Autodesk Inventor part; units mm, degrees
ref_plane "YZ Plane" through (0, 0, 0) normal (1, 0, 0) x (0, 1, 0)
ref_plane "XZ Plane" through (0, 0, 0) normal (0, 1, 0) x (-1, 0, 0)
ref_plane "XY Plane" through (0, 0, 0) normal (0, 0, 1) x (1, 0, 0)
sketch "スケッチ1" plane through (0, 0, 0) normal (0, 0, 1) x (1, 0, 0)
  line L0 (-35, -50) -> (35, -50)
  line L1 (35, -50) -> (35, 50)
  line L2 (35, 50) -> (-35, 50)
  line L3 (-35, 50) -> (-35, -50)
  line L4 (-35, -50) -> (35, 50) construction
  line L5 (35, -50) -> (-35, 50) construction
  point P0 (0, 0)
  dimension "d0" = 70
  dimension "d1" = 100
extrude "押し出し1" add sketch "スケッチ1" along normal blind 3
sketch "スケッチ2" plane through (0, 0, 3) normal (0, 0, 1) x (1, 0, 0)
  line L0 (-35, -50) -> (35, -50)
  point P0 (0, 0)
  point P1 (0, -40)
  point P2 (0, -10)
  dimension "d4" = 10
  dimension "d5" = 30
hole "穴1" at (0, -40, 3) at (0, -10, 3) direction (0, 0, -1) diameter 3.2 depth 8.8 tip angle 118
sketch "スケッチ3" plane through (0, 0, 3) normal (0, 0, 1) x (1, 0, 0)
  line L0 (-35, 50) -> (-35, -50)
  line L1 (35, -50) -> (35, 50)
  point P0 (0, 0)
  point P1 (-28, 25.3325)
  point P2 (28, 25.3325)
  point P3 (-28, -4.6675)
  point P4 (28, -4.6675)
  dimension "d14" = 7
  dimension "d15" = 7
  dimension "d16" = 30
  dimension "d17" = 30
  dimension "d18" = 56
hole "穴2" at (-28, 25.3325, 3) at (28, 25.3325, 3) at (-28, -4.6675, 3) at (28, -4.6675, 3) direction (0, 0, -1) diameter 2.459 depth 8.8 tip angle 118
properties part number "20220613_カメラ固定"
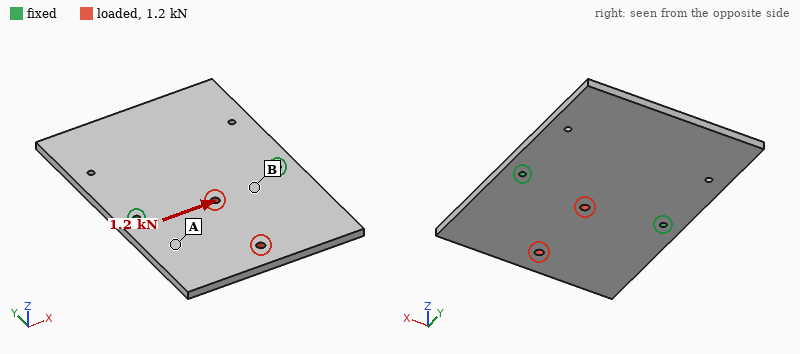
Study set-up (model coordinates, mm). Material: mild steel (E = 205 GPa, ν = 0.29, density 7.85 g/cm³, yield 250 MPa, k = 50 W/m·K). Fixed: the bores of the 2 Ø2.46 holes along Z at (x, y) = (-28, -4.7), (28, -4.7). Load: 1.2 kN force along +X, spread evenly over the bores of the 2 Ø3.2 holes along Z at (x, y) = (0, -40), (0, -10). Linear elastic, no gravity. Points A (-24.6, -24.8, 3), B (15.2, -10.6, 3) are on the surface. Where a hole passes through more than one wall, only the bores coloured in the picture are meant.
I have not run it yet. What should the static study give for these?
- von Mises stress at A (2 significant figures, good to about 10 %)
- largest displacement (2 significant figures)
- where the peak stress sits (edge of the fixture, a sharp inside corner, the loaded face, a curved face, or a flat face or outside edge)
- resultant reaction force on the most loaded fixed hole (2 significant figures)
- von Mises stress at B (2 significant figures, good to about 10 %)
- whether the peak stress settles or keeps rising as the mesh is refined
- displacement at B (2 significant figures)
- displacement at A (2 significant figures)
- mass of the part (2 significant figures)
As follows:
4.9 MPa
3.7 µm
edge of the fixture
740 N
10 MPa
keeps rising
1.1 µm
2.1 µm
160 g
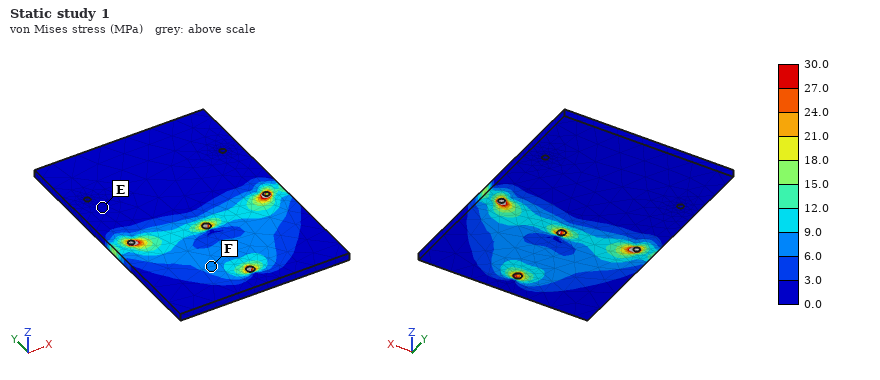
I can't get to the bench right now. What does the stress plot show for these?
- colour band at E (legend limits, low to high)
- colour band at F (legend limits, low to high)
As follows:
0.0 to 3.0 MPa
6.0 to 9.0 MPa
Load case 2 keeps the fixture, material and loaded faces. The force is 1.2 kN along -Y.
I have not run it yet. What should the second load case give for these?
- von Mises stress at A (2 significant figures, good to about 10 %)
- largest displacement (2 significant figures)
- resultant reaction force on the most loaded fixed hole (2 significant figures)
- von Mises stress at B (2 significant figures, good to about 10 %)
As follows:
5.0 MPa
2.5 µm
600 N
5.8 MPa
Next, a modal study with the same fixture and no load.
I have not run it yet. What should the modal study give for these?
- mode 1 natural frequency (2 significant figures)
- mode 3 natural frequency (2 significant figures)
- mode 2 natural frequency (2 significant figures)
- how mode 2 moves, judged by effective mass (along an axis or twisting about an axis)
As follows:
650 Hz
1700 Hz
1100 Hz
along Z
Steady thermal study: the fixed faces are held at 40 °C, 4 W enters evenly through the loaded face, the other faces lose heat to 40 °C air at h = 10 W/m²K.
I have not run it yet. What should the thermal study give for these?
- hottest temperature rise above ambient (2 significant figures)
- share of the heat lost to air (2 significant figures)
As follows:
16 K
22 %
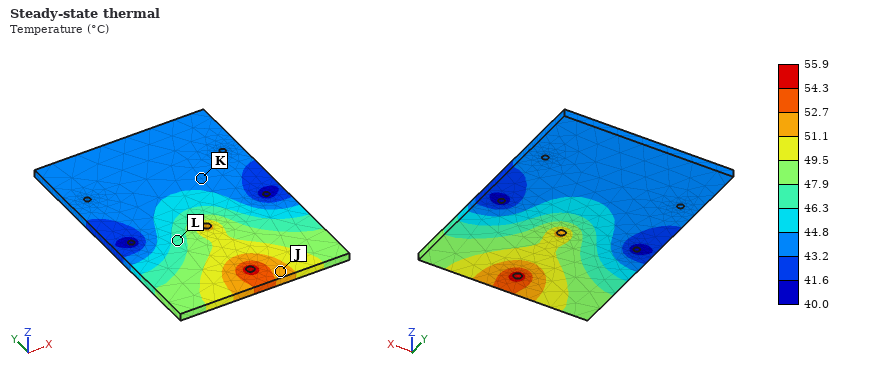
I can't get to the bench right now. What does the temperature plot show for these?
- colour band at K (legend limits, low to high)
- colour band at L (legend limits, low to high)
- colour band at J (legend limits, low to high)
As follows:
43.2 to 44.8 °C
46.3 to 47.9 °C
51.1 to 52.7 °C
